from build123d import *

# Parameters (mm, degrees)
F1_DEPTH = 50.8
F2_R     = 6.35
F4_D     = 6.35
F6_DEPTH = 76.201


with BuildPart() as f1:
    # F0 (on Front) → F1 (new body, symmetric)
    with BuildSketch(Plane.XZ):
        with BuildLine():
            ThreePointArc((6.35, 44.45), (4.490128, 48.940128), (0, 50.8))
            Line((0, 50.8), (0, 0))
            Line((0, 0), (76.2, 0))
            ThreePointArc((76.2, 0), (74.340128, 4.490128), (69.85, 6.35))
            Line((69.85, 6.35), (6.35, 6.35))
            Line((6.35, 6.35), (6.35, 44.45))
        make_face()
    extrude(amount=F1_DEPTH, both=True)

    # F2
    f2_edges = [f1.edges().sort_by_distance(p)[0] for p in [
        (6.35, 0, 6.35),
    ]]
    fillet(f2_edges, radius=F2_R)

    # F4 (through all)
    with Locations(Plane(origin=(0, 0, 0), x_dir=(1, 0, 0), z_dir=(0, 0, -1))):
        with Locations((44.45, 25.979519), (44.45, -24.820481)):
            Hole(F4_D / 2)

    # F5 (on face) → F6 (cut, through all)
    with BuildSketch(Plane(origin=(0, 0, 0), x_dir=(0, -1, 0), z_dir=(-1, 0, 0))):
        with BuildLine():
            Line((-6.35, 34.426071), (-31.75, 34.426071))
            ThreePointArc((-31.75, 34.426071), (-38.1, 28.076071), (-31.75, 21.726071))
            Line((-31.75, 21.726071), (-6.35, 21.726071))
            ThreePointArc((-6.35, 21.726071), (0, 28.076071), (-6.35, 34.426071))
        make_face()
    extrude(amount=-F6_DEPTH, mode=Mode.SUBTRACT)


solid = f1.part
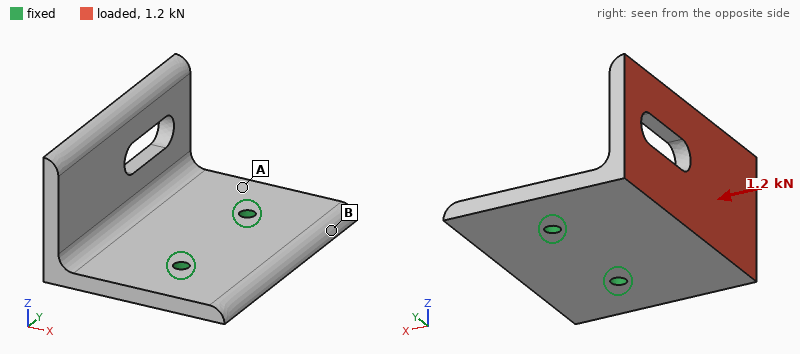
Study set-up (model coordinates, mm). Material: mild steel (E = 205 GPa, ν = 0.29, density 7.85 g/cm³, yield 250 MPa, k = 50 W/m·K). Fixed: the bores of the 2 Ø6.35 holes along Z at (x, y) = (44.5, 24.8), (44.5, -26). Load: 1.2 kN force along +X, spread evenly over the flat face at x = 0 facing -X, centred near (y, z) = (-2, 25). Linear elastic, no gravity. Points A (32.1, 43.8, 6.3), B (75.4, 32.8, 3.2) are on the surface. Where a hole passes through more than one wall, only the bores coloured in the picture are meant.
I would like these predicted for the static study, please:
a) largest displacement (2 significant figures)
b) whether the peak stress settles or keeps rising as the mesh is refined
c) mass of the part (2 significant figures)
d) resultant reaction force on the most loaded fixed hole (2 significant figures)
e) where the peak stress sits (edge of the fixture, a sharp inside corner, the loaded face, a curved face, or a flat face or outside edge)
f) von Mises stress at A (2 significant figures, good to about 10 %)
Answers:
0.16 mm
keeps rising
580 g
630 N
edge of the fixture
33 MPa
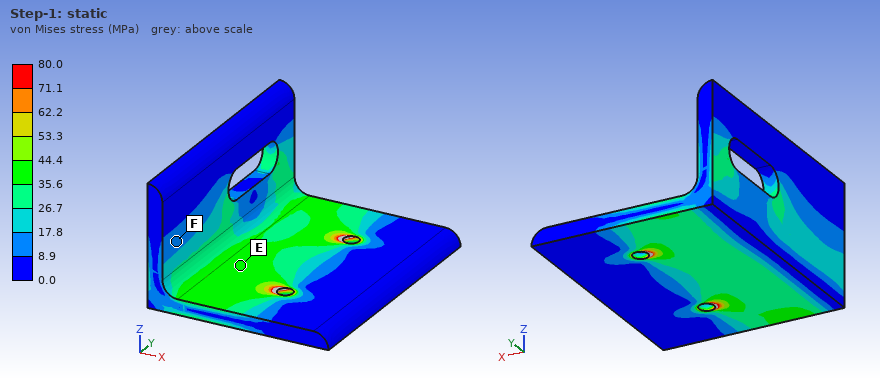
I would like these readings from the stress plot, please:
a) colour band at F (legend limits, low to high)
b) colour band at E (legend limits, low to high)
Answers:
8.9 to 17.8 MPa
35.6 to 44.4 MPa
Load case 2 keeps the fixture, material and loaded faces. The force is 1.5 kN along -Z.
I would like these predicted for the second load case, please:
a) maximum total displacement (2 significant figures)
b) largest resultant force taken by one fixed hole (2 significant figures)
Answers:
0.21 mm
780 N
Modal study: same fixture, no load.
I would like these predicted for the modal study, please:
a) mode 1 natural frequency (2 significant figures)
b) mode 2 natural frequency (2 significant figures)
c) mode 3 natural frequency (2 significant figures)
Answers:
910 Hz
1500 Hz
2500 Hz
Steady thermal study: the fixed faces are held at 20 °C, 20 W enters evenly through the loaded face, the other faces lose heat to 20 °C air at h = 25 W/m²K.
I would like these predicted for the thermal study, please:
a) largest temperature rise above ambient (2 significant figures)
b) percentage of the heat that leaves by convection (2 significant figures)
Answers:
35 K
35 %
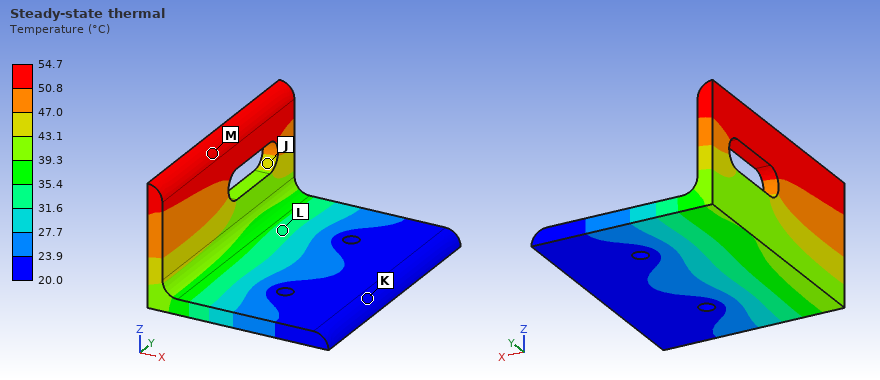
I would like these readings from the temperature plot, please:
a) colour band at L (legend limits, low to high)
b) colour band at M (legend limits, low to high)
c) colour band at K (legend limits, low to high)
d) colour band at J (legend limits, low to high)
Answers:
31.6 to 35.4 °C
50.8 to 54.7 °C
20.0 to 23.9 °C
43.1 to 47.0 °C
